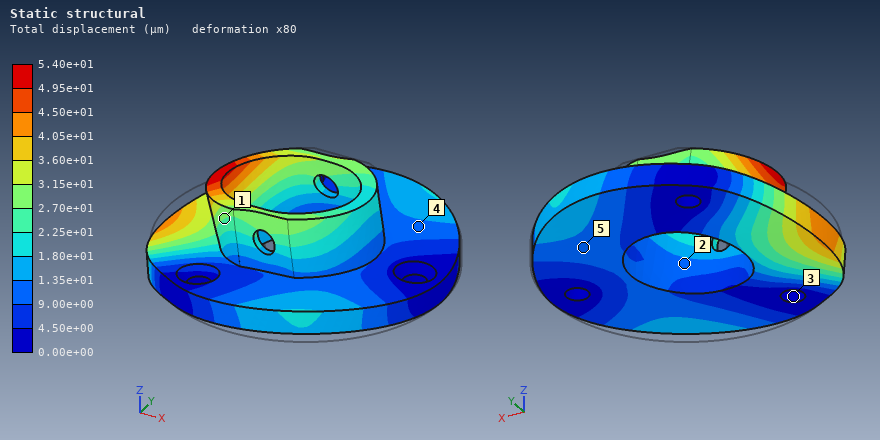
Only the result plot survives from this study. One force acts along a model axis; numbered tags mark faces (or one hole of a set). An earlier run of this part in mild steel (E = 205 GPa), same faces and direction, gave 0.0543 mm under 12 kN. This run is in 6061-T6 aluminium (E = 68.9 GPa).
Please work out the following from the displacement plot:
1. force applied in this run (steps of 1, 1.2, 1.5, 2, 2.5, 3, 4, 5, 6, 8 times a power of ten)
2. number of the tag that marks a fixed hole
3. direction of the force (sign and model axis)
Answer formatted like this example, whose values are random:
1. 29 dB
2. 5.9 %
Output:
1. 4 kN
2. 3
3. -X
